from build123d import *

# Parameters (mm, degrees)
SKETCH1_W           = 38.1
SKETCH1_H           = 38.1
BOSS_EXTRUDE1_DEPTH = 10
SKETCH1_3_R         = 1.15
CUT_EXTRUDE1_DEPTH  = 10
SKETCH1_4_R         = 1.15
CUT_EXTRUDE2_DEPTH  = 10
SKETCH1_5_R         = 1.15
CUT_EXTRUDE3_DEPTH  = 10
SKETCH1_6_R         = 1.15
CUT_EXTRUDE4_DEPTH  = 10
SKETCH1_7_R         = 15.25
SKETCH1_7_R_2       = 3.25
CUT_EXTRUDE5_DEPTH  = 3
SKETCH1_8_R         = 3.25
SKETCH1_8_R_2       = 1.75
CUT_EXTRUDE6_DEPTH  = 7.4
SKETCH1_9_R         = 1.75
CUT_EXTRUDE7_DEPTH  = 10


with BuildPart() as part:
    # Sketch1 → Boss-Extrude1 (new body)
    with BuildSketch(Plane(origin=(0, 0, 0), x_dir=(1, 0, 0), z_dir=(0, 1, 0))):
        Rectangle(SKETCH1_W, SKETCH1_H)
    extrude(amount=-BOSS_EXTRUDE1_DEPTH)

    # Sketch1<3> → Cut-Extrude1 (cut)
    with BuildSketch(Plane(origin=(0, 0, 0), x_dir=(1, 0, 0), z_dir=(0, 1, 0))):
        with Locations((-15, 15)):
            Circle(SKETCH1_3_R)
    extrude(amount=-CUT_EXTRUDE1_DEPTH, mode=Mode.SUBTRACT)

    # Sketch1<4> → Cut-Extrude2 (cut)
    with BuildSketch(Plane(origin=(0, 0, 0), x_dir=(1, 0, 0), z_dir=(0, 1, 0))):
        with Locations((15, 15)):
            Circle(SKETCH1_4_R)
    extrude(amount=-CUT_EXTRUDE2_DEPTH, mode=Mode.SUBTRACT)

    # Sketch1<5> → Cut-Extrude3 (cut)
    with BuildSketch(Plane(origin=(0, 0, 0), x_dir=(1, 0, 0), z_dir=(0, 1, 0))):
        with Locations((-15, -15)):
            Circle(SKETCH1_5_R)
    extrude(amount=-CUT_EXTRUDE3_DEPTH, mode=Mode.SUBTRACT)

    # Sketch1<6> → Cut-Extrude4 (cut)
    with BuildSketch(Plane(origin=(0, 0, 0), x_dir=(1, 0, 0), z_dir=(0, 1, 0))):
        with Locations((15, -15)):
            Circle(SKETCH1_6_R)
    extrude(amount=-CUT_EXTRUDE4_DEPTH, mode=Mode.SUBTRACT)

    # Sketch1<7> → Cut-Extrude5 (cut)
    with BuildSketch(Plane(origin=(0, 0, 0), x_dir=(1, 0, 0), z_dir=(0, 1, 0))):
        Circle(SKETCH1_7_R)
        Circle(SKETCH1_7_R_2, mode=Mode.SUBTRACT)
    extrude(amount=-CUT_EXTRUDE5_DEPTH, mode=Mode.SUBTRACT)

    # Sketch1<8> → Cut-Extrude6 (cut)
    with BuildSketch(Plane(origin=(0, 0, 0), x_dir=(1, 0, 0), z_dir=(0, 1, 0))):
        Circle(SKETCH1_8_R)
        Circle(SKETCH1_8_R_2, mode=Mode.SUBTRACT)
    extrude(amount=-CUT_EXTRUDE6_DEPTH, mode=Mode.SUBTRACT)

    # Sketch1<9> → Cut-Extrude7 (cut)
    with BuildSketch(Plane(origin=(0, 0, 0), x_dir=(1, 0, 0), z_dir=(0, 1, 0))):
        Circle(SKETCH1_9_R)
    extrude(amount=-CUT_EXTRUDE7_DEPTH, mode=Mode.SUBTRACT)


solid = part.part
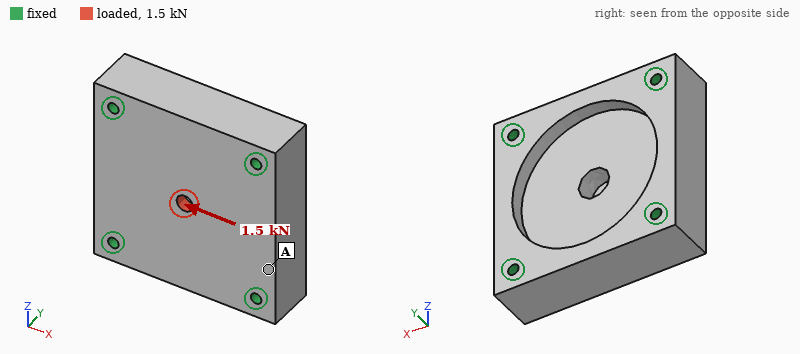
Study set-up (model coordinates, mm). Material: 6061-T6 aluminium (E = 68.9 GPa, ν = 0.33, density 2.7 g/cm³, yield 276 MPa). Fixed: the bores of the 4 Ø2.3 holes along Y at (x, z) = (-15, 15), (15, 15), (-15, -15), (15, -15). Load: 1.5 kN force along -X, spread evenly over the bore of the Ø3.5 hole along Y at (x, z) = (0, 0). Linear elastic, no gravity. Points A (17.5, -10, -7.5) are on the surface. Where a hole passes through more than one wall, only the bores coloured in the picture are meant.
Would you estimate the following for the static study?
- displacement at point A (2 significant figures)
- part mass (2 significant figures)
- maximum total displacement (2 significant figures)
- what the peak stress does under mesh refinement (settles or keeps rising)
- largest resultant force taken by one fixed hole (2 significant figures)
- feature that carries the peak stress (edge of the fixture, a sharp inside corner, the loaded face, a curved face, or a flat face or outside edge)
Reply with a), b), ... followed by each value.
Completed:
a) 1.1 µm
b) 32 g
c) 4.9 µm
d) keeps rising
e) 430 N
f) a sharp inside corner
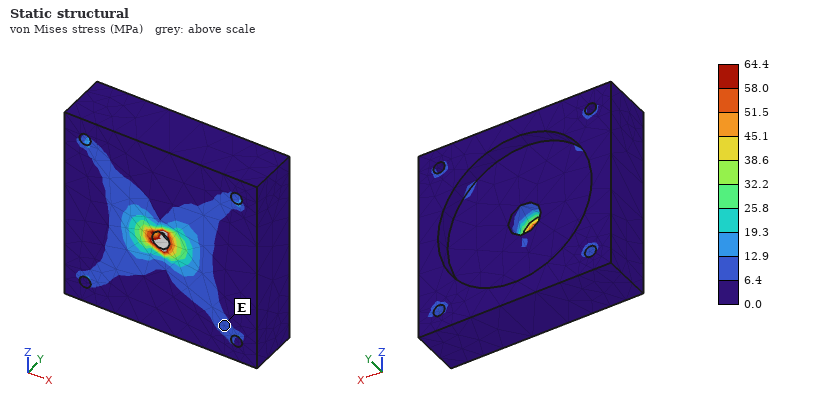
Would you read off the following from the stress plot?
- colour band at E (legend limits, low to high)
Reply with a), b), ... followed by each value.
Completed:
a) 6.4 to 12.9 MPa
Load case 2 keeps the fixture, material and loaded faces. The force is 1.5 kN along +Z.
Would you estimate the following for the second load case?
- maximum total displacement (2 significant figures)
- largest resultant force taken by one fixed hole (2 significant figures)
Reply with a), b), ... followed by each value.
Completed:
a) 4.9 µm
b) 430 N
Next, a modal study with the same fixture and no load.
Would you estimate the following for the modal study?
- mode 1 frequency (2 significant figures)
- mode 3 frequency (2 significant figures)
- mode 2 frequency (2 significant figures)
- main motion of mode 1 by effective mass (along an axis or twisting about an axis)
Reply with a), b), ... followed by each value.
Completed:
a) 25 kHz
b) 36 kHz
c) 36 kHz
d) along Y
